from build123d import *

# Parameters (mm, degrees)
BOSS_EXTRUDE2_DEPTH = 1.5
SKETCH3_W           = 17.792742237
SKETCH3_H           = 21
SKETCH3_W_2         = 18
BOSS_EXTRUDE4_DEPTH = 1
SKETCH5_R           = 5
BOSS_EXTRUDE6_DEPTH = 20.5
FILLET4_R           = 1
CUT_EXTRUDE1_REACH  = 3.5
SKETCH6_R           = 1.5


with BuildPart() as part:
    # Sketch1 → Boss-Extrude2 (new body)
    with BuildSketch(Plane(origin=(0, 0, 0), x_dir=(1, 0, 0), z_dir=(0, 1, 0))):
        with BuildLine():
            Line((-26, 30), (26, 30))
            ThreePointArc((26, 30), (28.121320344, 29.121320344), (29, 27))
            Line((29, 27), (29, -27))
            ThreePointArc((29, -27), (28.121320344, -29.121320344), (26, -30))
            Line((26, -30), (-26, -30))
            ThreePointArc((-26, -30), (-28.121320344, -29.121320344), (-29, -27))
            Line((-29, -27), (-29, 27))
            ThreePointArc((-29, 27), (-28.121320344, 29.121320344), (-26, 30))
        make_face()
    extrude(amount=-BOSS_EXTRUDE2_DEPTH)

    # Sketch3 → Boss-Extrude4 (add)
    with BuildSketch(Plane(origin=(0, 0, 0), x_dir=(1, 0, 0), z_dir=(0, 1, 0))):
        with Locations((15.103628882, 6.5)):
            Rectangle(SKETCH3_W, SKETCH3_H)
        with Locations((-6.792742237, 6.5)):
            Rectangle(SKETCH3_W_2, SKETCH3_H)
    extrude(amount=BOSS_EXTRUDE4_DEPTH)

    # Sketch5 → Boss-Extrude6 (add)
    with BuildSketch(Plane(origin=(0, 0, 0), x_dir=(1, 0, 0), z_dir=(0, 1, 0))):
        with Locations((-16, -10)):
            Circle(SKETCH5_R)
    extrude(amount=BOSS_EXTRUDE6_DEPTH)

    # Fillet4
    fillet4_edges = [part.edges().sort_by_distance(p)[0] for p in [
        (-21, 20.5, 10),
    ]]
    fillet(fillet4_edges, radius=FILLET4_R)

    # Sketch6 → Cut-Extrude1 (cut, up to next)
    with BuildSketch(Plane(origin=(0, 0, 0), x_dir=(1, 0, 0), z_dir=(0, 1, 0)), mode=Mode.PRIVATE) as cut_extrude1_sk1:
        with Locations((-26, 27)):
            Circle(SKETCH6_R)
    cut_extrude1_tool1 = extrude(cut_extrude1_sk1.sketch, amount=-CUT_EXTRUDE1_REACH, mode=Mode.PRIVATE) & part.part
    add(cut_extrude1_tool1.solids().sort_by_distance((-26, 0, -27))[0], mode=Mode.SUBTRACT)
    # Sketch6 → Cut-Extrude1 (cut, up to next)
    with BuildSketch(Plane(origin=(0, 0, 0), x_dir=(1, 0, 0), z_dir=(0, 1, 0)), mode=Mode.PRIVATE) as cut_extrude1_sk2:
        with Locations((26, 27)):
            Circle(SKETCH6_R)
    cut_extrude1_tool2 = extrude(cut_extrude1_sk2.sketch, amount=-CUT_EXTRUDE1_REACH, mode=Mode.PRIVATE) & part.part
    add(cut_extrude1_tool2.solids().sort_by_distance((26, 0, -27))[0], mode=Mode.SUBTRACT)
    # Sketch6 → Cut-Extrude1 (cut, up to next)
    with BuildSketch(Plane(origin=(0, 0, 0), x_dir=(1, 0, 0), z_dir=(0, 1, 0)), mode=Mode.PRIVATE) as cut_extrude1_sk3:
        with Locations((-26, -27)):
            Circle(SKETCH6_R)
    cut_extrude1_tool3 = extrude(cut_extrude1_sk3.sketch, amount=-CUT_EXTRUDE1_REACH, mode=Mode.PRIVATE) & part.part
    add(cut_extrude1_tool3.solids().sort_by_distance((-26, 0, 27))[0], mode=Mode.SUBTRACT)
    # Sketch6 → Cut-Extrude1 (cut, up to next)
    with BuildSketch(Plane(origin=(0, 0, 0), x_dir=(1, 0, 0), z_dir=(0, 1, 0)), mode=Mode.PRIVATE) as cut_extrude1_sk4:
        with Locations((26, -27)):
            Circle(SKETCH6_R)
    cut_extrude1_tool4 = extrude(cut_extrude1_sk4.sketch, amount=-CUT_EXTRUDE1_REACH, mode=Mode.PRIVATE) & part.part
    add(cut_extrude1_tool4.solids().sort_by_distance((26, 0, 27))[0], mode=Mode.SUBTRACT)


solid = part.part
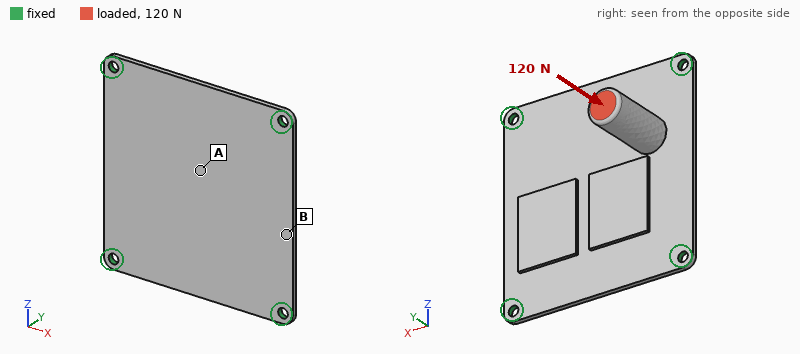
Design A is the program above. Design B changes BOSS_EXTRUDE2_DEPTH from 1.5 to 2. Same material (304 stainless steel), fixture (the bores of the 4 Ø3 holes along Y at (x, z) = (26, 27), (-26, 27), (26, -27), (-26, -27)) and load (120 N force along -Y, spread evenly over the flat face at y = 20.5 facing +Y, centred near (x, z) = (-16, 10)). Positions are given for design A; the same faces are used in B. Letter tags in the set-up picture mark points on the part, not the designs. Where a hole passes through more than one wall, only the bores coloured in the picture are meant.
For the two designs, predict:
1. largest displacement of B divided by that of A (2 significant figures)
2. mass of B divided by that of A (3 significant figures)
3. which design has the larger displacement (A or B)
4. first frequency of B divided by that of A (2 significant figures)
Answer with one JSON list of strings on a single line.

["0.48", "1.23", "A", "1.4"]
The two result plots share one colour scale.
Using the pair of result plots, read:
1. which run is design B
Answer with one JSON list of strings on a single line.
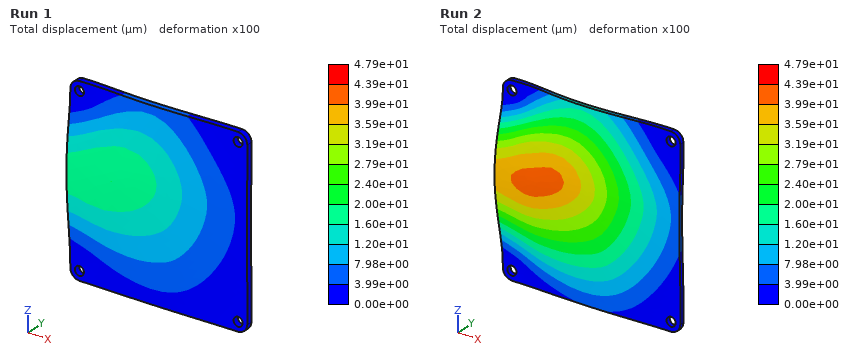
["Run 1"]
